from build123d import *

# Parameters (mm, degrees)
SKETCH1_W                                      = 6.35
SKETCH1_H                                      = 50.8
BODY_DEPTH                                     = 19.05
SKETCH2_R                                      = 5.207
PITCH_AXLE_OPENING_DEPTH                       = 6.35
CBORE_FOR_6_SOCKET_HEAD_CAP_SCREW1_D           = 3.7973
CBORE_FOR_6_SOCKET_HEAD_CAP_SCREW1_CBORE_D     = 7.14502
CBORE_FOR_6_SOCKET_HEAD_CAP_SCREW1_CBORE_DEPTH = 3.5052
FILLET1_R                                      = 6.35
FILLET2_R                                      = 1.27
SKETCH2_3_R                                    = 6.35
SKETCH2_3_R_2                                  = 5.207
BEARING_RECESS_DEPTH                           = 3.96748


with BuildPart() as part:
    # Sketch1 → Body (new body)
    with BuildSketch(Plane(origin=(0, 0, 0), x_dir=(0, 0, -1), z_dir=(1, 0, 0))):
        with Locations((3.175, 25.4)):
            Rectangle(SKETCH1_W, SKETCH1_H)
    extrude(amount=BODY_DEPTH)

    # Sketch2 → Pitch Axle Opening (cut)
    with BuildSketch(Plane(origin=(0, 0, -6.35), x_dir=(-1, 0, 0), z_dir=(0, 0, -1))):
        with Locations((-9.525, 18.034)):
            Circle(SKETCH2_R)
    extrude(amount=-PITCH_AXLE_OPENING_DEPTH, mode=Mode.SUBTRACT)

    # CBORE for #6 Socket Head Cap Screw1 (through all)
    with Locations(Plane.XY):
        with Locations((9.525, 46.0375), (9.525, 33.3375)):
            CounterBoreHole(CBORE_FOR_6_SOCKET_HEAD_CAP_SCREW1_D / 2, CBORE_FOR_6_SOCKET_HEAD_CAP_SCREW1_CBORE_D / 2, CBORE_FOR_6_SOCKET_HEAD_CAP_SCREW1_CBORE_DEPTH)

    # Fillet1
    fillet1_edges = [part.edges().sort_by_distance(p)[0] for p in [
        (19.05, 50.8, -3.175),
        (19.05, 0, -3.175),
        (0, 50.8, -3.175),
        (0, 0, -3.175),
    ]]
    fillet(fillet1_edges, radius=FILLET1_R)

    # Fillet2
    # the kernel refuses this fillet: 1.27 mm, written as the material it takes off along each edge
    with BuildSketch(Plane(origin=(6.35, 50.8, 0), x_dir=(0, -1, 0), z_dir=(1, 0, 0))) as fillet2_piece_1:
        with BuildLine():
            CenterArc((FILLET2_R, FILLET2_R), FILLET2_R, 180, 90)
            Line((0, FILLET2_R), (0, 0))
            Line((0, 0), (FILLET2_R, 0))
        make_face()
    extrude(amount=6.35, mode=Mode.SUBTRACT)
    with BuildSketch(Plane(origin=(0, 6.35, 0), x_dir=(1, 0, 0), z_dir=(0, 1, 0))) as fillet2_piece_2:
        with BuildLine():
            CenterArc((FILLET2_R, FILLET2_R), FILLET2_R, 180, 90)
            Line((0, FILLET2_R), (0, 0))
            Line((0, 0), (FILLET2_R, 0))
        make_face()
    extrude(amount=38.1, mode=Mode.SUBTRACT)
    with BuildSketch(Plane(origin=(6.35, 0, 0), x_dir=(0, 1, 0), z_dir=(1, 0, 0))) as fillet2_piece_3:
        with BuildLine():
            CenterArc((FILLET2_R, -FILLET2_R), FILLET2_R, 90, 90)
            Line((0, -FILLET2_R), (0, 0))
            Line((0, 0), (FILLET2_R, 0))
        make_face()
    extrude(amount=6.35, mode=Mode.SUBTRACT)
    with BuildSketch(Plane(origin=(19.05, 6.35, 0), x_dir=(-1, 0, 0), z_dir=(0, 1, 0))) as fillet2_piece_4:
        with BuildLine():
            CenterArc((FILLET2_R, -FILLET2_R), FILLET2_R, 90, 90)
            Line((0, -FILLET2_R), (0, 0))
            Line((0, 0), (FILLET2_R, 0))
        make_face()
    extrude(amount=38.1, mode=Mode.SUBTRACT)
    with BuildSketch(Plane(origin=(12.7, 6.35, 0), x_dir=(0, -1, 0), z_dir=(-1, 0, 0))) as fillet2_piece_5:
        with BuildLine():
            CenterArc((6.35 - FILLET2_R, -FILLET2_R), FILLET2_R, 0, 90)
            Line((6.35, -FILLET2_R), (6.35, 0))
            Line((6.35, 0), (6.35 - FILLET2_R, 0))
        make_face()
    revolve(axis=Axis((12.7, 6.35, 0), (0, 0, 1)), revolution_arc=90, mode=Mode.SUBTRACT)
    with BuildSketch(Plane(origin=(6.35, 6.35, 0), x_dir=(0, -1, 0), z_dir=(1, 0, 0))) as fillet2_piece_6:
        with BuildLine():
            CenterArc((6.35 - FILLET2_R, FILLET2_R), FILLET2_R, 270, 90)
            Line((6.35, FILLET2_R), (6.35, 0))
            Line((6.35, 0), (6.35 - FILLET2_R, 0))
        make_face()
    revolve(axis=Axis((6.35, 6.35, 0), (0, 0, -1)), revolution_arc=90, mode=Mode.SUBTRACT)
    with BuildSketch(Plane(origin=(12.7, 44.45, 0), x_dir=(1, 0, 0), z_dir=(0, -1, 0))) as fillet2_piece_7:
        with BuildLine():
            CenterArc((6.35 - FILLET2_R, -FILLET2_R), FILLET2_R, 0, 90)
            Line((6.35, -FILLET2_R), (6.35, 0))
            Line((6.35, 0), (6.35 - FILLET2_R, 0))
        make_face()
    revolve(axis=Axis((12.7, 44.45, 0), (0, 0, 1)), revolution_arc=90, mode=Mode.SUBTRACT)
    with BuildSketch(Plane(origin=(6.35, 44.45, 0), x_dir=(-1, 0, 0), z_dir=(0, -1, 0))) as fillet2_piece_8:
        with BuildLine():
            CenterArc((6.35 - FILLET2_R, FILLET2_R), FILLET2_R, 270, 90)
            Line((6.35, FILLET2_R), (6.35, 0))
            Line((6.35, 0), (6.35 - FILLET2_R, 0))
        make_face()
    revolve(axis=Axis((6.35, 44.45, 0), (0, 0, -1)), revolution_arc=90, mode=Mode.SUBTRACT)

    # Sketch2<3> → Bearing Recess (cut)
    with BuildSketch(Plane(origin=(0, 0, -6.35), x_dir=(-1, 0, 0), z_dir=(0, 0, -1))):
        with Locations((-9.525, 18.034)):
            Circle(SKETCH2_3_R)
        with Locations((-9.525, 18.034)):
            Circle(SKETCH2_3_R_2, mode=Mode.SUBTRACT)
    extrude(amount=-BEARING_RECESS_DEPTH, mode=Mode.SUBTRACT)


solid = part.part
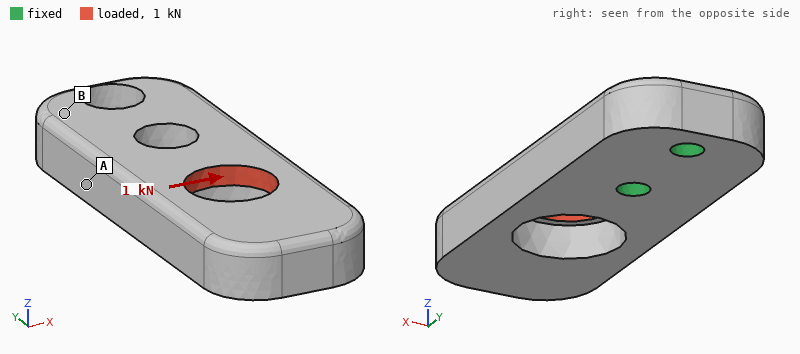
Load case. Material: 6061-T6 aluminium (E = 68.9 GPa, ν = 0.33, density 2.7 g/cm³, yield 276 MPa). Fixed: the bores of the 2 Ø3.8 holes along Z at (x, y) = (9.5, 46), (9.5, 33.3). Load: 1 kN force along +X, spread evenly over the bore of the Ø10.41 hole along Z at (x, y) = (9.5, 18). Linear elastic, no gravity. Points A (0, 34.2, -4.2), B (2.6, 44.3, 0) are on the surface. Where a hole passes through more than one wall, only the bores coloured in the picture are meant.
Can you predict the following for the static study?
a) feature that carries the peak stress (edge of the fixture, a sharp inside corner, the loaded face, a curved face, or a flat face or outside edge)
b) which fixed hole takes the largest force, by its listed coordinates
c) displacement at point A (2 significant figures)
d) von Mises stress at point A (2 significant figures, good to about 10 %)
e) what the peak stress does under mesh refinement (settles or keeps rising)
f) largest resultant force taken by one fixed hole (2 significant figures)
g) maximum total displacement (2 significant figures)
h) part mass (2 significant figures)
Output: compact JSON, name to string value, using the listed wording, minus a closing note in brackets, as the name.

{"feature that carries the peak stress": "edge of the fixture", "which fixed hole takes the largest force, by its listed coordinates": "(9.5, 33.3)", "displacement at point A": "15 µm", "von Mises stress at point A": "46 MPa", "what the peak stress does under mesh refinement": "keeps rising", "largest resultant force taken by one fixed hole": "1.8 kN", "maximum total displacement": "75 µm", "part mass": "13 g"}
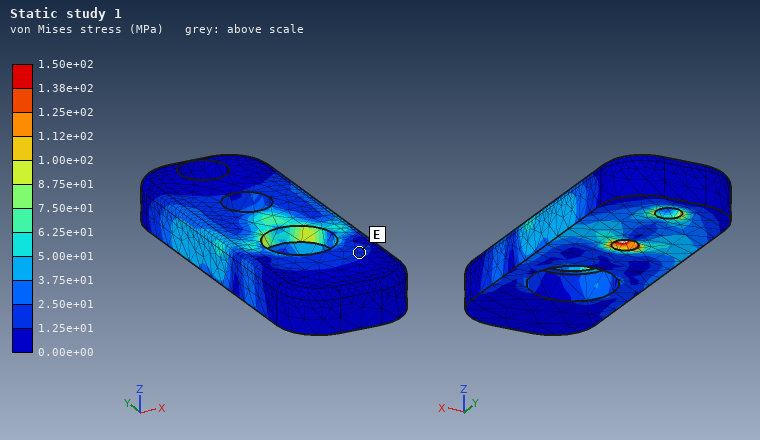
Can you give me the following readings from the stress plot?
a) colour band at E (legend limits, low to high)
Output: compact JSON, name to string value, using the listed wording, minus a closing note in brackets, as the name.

{"colour band at E": "1.25e+01 to 2.50e+01 MPa"}
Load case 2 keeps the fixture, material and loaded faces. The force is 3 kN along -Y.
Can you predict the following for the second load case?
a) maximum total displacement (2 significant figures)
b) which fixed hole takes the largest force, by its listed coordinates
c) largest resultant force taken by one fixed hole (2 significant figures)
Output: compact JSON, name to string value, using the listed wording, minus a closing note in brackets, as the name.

{"maximum total displacement": "0.18 mm", "which fixed hole takes the largest force, by its listed coordinates": "(9.5, 33.3)", "largest resultant force taken by one fixed hole": "1.8 kN"}
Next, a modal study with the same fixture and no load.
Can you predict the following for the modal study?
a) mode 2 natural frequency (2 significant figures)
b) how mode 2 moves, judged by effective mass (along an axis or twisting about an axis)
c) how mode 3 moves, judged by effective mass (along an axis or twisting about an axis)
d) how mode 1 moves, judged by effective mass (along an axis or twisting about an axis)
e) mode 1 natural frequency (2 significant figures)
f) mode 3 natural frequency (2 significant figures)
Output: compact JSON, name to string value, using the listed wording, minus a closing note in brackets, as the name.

{"mode 2 natural frequency": "7200 Hz", "how mode 2 moves, judged by effective mass": "along X", "how mode 3 moves, judged by effective mass": "twisting about Y", "how mode 1 moves, judged by effective mass": "along Z", "mode 1 natural frequency": "3500 Hz", "mode 3 natural frequency": "9400 Hz"}
